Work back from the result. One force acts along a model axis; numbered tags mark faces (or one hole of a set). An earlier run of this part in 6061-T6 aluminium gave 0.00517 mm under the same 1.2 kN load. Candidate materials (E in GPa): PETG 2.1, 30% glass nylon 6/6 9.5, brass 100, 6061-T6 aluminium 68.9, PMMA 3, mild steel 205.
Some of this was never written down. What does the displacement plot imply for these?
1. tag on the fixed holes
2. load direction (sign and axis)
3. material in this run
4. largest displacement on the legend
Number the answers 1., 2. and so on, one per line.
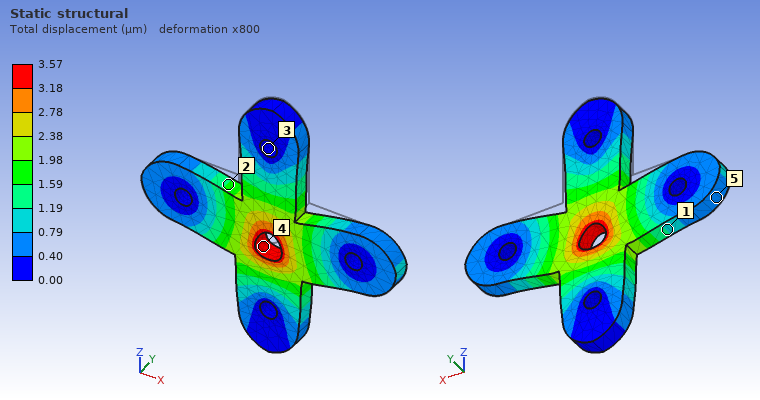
1. 3
2. -Z
3. brass
4. 3.57 µm
